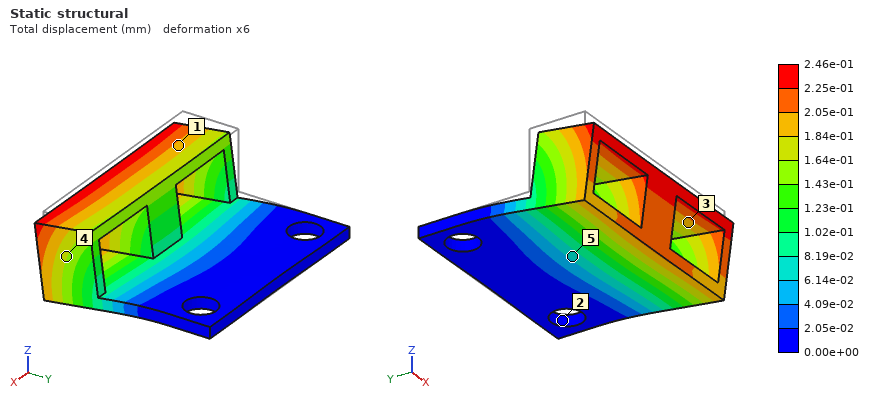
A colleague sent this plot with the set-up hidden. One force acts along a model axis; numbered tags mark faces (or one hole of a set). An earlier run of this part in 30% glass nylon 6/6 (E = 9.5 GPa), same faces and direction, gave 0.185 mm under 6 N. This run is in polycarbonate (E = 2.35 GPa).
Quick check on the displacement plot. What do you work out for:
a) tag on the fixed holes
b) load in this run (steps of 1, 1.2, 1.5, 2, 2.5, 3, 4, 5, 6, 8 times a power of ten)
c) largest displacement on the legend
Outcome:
2
2 N
2.46e-01 mm
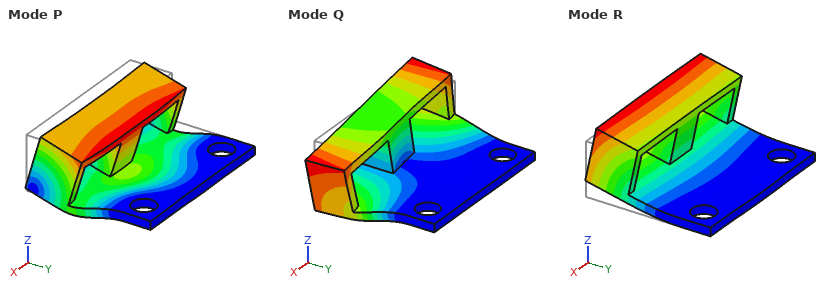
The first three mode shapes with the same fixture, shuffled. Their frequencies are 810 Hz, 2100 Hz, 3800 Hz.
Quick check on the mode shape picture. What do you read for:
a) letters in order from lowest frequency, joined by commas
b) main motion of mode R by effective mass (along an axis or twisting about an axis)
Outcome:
R, Q, P
along Z
